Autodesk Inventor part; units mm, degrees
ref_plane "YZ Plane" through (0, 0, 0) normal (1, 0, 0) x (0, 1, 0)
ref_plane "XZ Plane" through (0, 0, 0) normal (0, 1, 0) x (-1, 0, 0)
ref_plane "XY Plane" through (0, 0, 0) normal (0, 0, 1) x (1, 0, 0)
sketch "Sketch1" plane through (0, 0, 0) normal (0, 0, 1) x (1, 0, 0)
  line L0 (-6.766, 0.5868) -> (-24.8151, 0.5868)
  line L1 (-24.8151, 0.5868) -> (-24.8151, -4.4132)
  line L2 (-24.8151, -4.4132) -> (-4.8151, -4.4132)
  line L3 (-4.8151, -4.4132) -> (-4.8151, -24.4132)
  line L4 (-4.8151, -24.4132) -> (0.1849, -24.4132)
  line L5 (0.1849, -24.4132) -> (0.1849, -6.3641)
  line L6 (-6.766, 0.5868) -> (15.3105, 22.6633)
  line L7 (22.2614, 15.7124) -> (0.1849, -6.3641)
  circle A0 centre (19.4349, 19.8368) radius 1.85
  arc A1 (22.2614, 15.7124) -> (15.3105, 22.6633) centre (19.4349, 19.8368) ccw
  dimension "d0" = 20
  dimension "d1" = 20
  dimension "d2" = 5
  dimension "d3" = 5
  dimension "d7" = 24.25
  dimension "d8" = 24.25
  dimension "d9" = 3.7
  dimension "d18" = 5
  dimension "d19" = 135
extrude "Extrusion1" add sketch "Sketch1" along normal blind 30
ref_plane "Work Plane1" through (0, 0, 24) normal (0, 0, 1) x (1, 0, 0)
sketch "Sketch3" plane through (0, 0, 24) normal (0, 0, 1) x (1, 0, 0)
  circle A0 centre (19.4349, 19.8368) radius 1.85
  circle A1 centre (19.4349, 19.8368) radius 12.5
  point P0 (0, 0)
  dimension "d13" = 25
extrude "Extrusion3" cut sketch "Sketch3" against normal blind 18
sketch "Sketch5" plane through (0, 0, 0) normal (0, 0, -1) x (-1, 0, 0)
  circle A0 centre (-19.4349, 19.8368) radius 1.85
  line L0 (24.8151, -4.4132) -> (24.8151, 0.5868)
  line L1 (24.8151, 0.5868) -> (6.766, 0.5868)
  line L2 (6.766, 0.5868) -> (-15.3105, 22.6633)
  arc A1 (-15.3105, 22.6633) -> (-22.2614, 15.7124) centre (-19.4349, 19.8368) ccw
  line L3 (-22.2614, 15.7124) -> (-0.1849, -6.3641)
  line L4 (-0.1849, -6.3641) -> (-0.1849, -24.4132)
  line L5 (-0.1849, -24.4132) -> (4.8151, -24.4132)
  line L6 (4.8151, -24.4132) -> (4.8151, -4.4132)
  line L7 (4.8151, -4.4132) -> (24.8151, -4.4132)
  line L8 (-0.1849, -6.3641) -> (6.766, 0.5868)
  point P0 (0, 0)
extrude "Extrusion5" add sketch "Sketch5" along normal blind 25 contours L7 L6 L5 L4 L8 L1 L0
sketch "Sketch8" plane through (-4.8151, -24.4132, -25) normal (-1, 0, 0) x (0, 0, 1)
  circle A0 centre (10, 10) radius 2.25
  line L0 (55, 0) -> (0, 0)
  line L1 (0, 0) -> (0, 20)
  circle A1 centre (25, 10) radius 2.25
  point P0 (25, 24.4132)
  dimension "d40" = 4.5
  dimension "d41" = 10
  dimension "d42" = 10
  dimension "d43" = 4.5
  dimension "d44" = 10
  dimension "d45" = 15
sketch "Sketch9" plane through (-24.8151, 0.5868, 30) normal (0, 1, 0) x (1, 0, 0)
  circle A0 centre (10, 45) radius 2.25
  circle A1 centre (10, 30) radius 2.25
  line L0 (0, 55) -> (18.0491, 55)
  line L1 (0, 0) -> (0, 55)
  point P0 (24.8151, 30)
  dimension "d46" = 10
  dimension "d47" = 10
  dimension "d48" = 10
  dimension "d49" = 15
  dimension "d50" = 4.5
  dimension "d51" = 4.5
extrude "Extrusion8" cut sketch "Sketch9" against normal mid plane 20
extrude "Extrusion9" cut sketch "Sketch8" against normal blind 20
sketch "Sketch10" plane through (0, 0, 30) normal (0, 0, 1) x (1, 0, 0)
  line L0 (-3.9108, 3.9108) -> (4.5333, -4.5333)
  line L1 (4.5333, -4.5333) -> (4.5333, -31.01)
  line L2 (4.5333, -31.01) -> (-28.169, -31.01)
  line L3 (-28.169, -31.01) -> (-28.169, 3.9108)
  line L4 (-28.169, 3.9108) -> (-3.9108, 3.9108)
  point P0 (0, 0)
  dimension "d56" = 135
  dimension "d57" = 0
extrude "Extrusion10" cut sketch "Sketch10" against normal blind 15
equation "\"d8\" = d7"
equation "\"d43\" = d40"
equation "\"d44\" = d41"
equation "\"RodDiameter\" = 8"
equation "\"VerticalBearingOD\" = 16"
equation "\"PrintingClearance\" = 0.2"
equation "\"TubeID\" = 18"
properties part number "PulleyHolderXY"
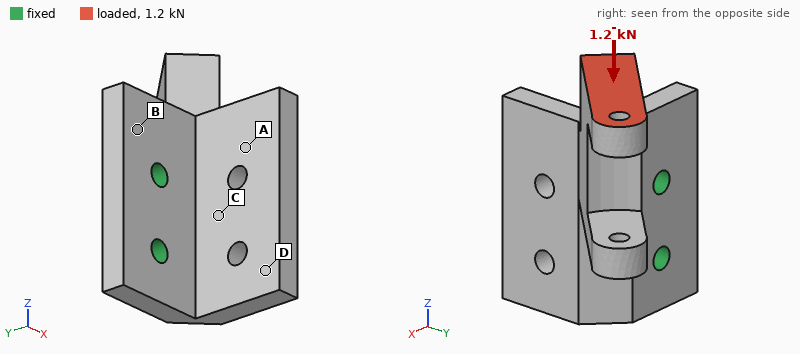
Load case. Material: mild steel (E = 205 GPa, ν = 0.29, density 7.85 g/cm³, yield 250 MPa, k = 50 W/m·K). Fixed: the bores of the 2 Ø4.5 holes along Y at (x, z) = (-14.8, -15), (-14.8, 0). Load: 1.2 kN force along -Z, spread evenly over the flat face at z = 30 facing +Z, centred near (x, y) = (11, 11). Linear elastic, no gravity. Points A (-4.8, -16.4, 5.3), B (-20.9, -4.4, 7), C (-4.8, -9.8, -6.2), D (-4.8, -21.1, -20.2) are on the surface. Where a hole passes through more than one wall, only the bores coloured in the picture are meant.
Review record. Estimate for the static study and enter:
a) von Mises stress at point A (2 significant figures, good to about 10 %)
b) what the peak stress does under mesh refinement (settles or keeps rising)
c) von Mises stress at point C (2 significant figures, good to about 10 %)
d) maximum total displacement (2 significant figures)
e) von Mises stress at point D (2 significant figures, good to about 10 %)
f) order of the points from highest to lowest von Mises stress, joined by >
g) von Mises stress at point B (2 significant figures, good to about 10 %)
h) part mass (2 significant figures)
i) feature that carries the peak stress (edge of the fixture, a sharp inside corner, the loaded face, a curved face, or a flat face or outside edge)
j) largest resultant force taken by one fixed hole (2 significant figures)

27 MPa
keeps rising
45 MPa
0.12 mm
12 MPa
B > C > A > D
66 MPa
120 g
edge of the fixture
1.6 kN
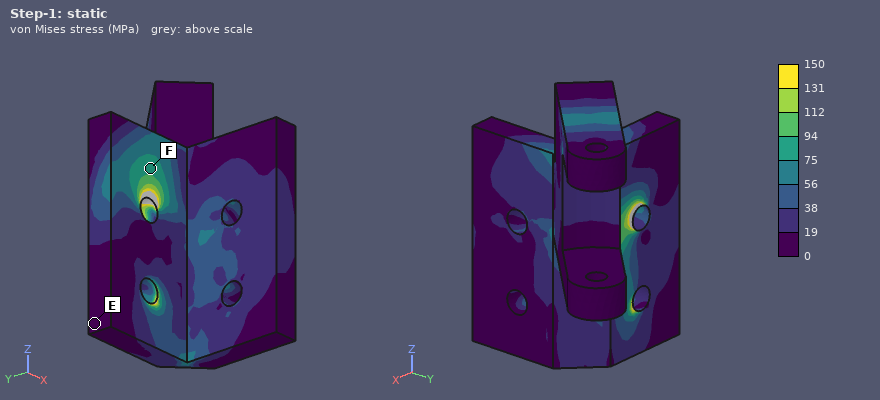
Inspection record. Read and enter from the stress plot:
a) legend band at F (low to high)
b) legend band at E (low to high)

75 to 94 MPa
0 to 19 MPa
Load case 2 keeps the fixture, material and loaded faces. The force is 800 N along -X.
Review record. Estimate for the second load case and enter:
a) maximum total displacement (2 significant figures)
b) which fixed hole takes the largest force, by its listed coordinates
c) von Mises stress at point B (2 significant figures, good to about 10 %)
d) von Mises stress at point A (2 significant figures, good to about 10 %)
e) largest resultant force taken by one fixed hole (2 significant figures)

0.14 mm
(-14.8, 0)
19 MPa
23 MPa
2.0 kN
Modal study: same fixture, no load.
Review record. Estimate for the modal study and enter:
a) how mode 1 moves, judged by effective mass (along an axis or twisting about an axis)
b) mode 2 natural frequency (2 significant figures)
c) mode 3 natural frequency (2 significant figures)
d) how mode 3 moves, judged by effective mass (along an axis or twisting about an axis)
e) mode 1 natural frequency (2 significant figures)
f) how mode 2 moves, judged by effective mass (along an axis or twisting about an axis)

along Y
3300 Hz
5200 Hz
along X
1700 Hz
along Z
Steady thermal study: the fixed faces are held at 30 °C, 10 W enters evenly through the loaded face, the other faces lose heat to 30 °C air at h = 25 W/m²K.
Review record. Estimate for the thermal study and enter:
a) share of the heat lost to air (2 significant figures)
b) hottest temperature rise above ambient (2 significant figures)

29 %
62 K
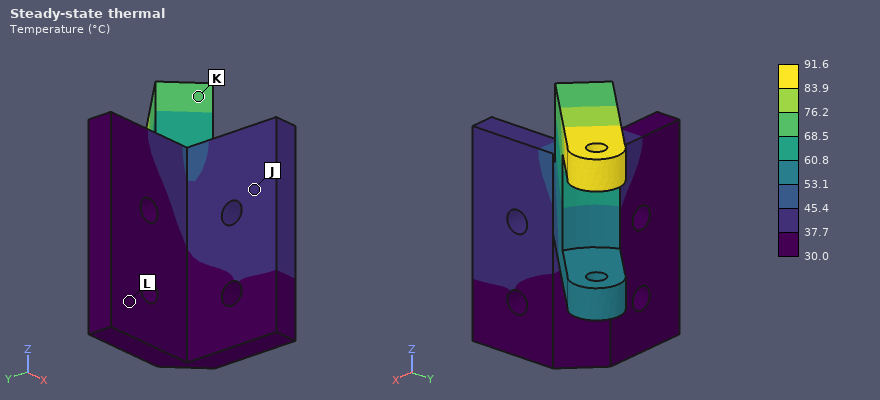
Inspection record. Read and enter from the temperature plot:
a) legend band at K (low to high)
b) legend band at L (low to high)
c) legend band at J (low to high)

68.5 to 76.2 °C
30.0 to 37.7 °C
37.7 to 45.4 °C
